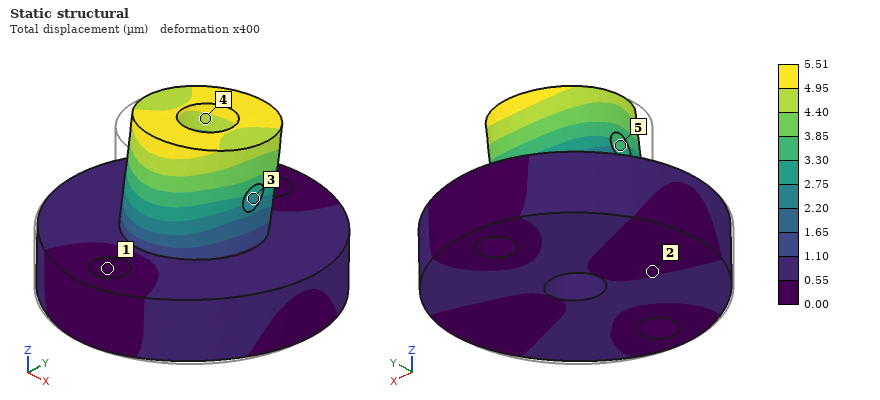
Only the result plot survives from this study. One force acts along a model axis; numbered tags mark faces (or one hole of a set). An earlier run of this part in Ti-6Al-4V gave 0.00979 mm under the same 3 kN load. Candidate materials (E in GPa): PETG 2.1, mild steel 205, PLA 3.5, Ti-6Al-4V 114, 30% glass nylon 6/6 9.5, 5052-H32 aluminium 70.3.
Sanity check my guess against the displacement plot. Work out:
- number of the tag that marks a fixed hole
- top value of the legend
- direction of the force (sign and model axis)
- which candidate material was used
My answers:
1
5.51 µm
+Y
mild steel
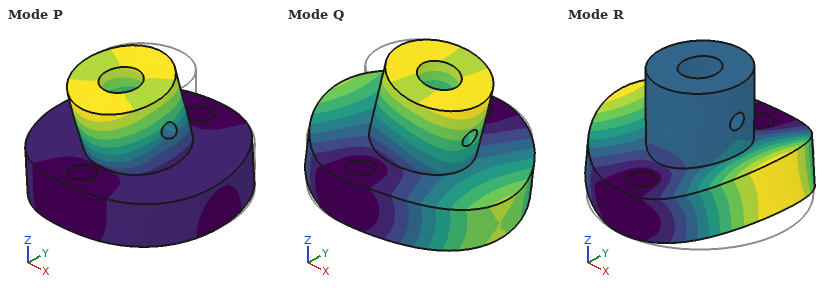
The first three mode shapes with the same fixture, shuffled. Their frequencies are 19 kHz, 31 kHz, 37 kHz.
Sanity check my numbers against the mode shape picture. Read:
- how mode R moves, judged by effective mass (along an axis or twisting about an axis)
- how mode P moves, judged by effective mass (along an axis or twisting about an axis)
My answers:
along Z
along Y
